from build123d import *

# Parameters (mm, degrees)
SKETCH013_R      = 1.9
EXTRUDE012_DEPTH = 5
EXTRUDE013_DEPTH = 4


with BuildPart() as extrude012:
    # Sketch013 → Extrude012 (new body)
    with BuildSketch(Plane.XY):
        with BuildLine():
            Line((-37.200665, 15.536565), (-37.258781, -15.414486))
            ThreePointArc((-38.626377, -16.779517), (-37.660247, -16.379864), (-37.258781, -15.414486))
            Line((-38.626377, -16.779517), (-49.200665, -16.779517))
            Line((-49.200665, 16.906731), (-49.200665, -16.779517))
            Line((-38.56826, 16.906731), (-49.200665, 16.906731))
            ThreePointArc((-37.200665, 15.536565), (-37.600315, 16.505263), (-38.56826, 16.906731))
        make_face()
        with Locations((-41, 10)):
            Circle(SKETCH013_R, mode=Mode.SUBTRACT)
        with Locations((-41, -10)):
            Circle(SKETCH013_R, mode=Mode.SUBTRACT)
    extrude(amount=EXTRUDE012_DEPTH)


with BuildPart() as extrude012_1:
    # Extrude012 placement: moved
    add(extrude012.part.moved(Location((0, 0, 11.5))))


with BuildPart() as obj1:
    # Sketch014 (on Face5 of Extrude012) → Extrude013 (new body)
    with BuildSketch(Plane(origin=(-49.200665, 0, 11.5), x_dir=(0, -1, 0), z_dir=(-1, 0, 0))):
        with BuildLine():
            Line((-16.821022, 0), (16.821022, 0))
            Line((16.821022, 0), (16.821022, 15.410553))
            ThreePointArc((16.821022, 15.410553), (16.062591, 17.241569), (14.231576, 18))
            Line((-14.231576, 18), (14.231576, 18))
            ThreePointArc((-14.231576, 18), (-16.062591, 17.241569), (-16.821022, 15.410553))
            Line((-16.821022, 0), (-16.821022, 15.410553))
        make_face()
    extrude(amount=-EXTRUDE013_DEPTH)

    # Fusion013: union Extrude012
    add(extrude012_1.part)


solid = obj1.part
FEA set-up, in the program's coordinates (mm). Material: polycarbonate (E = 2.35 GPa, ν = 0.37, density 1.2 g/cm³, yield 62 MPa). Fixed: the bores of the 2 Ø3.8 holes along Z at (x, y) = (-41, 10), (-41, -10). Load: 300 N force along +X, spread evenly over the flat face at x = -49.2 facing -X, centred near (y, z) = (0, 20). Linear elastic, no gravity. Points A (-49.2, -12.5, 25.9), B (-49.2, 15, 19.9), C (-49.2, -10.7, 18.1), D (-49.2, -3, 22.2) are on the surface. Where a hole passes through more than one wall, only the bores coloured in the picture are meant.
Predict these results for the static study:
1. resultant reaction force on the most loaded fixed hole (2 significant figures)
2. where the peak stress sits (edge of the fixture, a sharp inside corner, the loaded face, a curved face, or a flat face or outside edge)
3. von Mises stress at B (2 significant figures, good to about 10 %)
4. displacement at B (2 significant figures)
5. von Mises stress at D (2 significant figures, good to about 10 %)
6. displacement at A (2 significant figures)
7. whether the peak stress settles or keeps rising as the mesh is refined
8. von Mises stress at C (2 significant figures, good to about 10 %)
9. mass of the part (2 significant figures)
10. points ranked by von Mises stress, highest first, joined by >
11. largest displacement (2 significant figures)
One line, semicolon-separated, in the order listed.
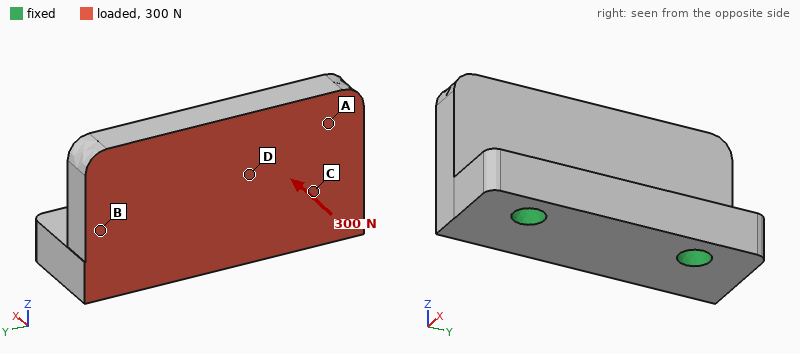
150 N; edge of the fixture; 8.9 MPa; 0.15 mm; 4.6 MPa; 0.32 mm; keeps rising; 12 MPa; 4.4 g; C > B > D > A; 0.44 mm
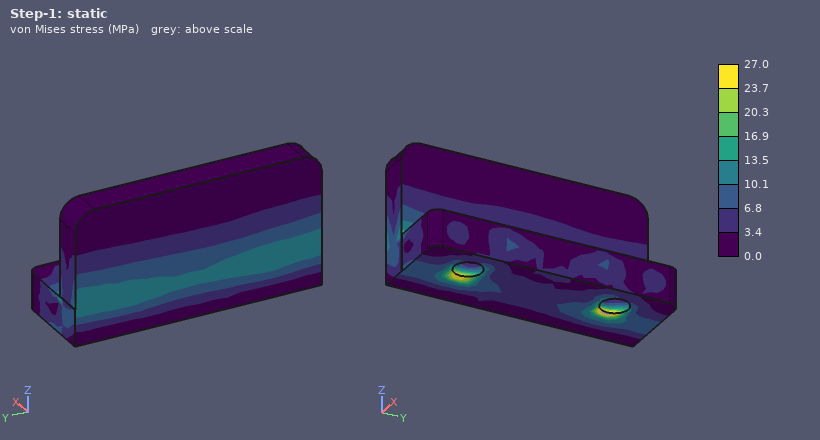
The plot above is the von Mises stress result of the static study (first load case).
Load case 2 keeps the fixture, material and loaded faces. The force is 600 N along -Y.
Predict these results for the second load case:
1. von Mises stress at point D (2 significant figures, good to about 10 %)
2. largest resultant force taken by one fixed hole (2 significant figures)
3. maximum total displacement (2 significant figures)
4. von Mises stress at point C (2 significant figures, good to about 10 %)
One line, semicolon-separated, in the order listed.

6.1 MPa; 390 N; 0.15 mm; 5.8 MPa
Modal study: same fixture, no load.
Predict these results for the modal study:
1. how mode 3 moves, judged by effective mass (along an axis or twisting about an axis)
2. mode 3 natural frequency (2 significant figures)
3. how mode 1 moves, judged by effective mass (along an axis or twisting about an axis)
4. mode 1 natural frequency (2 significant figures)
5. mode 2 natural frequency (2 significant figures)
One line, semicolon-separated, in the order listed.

along Y; 7000 Hz; along X; 3000 Hz; 4500 Hz
